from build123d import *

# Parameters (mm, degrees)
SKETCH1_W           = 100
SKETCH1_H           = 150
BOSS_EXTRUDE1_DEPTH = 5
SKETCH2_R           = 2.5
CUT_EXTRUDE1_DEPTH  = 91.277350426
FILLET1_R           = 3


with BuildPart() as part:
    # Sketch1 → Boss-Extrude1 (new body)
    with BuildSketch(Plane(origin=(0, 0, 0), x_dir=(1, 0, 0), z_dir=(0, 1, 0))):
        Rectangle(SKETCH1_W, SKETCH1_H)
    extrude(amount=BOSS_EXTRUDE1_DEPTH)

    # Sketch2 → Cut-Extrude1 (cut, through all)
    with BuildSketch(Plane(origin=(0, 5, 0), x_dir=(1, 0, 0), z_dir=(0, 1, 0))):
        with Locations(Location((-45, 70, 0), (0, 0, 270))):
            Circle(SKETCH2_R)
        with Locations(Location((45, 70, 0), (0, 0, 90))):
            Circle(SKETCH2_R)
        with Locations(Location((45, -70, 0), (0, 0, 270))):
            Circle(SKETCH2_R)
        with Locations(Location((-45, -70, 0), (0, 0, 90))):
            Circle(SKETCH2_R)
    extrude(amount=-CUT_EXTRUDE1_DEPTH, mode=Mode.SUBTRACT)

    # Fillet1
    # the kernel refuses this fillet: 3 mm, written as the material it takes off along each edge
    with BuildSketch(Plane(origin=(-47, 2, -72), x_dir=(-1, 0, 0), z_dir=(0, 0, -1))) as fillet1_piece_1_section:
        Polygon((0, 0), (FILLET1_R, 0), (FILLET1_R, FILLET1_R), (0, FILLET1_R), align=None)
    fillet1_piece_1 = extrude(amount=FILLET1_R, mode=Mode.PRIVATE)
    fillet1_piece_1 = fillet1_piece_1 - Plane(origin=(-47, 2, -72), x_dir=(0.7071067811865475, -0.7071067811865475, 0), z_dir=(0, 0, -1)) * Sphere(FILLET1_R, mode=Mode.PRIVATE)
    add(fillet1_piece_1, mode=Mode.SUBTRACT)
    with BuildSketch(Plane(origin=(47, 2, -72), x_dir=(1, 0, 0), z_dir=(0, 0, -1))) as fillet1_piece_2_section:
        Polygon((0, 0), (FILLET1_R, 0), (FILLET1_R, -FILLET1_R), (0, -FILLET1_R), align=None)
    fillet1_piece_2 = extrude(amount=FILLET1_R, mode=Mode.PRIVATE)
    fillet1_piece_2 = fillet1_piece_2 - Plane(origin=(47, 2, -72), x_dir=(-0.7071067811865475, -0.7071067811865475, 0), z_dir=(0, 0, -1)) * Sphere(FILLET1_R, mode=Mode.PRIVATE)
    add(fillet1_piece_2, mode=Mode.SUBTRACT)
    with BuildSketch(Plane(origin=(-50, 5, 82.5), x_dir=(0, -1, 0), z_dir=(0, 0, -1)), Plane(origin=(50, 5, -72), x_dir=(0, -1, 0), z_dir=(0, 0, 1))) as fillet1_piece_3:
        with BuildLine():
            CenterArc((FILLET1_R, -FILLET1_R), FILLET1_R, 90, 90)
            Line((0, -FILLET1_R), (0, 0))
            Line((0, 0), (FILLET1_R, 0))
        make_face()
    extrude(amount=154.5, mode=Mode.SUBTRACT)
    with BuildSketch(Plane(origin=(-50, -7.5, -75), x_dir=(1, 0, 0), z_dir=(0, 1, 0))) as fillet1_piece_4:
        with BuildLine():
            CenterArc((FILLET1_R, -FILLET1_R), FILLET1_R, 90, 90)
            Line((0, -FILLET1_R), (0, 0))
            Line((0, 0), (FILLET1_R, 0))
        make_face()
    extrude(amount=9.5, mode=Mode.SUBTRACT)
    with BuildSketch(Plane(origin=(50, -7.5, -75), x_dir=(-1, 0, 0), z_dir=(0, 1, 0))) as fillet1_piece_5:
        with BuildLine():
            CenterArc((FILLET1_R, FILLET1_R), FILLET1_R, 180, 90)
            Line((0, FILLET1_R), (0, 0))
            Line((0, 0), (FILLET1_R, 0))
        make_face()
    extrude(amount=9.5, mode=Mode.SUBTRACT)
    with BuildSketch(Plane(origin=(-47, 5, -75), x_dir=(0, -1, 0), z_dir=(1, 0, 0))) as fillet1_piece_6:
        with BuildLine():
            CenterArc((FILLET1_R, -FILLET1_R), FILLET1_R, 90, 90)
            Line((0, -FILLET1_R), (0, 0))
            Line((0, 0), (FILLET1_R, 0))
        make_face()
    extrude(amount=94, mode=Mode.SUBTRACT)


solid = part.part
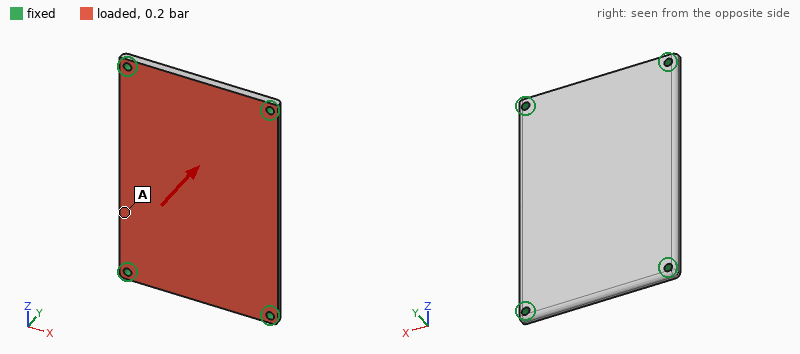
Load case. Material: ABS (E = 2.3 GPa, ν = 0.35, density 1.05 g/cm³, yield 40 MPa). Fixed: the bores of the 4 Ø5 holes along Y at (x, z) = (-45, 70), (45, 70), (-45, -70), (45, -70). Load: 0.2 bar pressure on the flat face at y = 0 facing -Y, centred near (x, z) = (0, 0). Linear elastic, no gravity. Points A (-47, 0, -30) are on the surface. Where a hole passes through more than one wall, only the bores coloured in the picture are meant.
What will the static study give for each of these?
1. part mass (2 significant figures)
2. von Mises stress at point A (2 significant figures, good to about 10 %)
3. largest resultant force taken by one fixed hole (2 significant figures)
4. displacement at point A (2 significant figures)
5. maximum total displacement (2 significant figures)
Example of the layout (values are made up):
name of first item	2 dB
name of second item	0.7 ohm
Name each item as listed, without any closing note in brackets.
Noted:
part mass	78 g
von Mises stress at point A	3.8 MPa
largest resultant force taken by one fixed hole	75 N
displacement at point A	0.95 mm
maximum total displacement	1.5 mm
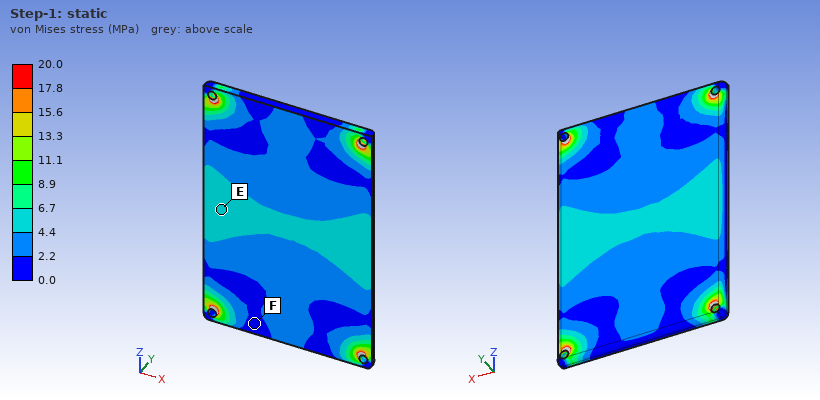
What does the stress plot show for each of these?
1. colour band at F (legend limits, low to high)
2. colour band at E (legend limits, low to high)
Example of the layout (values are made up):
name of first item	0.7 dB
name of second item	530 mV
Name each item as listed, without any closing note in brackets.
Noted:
colour band at F	0.0 to 2.2 MPa
colour band at E	4.4 to 6.7 MPa
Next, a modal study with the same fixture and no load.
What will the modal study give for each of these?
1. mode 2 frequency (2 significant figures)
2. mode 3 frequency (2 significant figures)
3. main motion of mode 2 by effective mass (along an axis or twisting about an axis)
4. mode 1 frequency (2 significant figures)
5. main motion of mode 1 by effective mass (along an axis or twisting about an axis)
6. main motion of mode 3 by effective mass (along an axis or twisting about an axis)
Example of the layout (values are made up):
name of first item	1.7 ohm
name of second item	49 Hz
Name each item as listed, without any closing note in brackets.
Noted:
mode 2 frequency	510 Hz
mode 3 frequency	750 Hz
main motion of mode 2 by effective mass	twisting about Z
mode 1 frequency	300 Hz
main motion of mode 1 by effective mass	along Y
main motion of mode 3 by effective mass	twisting about X
